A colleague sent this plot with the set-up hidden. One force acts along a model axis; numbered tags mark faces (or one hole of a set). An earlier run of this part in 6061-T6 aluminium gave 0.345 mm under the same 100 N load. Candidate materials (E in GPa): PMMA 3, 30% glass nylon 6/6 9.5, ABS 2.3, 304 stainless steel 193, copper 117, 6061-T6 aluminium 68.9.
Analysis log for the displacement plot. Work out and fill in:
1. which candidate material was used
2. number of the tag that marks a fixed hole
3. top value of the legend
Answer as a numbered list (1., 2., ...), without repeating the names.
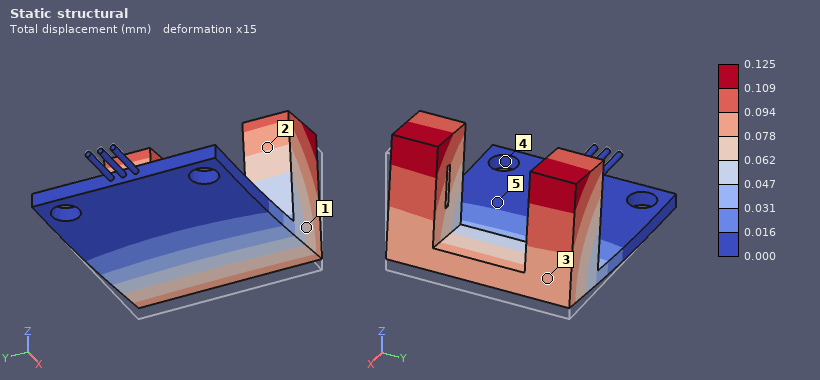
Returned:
1. 304 stainless steel
2. 4
3. 0.125 mm
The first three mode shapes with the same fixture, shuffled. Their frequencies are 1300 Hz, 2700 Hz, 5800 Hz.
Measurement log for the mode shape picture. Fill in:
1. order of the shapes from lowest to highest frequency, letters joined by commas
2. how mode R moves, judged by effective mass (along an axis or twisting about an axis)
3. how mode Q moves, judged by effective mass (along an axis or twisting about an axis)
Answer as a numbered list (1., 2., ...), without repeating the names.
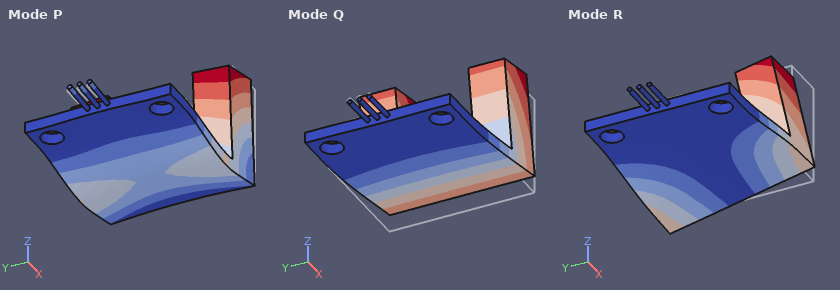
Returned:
1. Q, R, P
2. along Y
3. along Z
